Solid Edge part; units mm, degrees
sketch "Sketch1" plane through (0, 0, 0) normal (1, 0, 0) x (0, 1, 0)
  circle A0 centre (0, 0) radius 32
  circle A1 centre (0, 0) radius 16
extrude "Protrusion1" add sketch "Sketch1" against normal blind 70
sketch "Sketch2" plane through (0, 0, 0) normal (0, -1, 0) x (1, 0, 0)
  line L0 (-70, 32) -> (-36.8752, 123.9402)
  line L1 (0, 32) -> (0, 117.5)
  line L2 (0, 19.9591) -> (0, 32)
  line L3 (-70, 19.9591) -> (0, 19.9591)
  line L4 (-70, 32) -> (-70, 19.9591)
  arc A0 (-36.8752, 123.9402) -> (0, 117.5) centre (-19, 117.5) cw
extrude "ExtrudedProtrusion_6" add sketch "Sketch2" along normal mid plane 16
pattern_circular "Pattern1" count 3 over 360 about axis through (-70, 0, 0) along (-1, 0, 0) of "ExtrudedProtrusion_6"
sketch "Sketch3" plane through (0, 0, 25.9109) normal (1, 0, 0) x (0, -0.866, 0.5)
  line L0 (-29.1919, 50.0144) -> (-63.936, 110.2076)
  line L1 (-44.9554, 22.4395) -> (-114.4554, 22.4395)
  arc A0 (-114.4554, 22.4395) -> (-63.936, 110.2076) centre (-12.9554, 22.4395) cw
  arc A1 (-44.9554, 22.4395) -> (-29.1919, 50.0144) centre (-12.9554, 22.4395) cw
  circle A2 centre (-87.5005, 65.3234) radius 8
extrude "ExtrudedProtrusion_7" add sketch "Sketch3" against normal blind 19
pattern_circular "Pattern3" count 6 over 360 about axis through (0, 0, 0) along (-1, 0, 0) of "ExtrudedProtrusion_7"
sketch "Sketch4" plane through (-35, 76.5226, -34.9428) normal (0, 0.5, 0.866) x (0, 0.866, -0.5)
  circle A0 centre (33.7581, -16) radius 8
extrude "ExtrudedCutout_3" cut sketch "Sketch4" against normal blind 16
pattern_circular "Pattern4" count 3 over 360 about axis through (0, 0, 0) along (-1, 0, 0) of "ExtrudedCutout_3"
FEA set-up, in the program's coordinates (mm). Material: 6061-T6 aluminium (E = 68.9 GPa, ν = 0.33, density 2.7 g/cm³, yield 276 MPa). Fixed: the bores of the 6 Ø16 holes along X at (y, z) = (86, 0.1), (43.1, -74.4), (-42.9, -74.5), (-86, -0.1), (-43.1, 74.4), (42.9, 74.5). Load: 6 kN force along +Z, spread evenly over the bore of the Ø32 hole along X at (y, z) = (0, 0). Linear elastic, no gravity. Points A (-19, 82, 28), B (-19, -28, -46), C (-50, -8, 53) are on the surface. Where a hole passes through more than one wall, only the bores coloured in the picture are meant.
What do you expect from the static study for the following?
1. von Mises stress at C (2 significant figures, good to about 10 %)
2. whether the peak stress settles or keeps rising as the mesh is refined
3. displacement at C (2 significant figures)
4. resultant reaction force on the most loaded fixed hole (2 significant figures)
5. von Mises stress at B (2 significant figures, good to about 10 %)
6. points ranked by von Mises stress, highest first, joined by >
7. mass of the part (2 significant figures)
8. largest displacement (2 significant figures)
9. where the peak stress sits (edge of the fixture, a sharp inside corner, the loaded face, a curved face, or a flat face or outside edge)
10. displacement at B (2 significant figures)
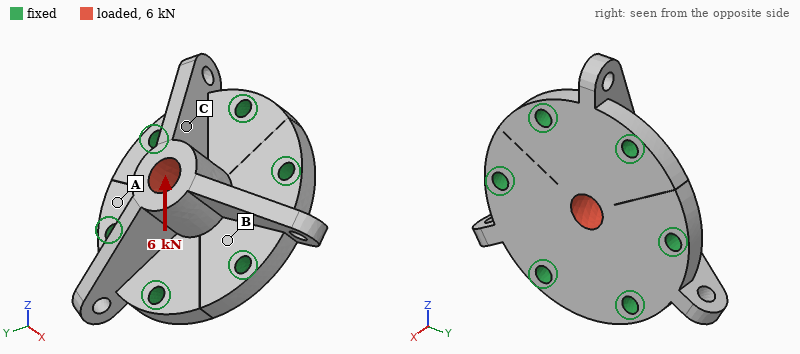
1.5 MPa
keeps rising
3.7 µm
1.5 kN
2.7 MPa
B > C > A
2.4 kg
7.7 µm
a sharp inside corner
1.2 µm
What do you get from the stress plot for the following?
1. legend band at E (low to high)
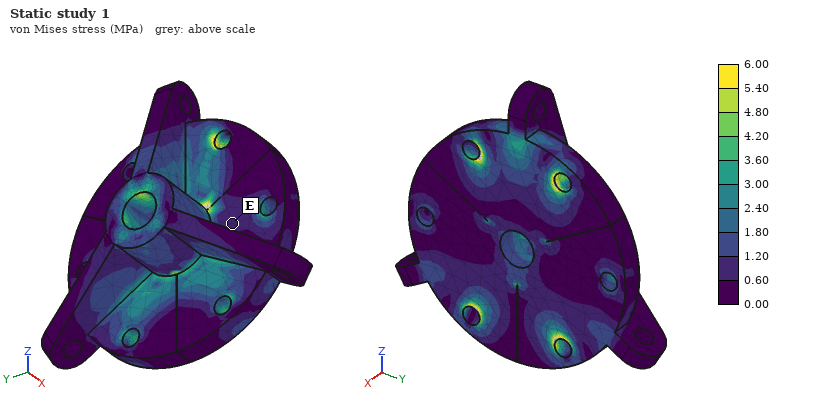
0.60 to 1.20 MPa
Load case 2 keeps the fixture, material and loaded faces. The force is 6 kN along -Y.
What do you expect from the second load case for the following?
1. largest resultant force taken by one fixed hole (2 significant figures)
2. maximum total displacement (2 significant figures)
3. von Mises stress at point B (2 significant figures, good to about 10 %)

1.8 kN
7.2 µm
1.4 MPa
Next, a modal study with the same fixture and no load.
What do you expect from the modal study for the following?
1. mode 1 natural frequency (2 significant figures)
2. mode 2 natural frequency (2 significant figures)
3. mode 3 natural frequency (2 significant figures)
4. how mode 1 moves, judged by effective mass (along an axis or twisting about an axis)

5000 Hz
5400 Hz
5400 Hz
along X
